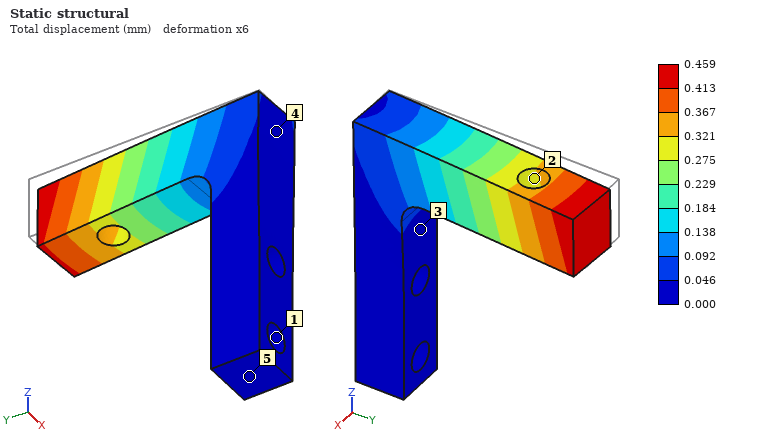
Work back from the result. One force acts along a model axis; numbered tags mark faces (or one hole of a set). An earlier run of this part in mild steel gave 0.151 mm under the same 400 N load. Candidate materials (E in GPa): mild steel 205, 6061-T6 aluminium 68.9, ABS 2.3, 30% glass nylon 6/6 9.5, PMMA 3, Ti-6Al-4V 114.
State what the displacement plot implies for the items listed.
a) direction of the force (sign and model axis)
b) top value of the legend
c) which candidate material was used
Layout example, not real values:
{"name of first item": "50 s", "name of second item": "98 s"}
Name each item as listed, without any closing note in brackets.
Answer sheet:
{"direction of the force": "+X", "top value of the legend": "0.459 mm", "which candidate material was used": "6061-T6 aluminium"}
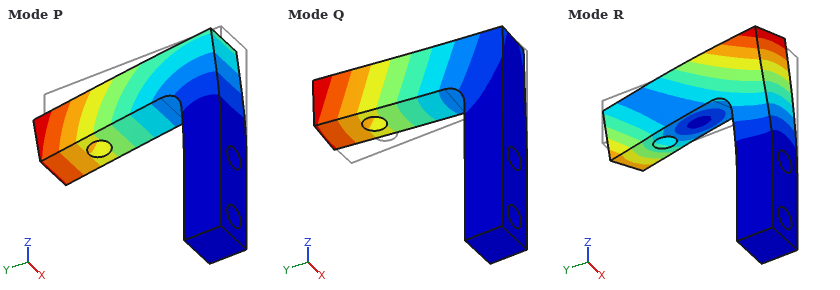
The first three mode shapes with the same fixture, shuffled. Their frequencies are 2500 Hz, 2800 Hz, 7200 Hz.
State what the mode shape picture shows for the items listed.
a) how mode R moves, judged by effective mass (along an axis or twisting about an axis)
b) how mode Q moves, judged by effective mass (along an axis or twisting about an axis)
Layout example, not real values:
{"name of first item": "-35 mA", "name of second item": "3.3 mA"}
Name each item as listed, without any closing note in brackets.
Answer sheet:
{"how mode R moves, judged by effective mass": "along X", "how mode Q moves, judged by effective mass": "along X"}
